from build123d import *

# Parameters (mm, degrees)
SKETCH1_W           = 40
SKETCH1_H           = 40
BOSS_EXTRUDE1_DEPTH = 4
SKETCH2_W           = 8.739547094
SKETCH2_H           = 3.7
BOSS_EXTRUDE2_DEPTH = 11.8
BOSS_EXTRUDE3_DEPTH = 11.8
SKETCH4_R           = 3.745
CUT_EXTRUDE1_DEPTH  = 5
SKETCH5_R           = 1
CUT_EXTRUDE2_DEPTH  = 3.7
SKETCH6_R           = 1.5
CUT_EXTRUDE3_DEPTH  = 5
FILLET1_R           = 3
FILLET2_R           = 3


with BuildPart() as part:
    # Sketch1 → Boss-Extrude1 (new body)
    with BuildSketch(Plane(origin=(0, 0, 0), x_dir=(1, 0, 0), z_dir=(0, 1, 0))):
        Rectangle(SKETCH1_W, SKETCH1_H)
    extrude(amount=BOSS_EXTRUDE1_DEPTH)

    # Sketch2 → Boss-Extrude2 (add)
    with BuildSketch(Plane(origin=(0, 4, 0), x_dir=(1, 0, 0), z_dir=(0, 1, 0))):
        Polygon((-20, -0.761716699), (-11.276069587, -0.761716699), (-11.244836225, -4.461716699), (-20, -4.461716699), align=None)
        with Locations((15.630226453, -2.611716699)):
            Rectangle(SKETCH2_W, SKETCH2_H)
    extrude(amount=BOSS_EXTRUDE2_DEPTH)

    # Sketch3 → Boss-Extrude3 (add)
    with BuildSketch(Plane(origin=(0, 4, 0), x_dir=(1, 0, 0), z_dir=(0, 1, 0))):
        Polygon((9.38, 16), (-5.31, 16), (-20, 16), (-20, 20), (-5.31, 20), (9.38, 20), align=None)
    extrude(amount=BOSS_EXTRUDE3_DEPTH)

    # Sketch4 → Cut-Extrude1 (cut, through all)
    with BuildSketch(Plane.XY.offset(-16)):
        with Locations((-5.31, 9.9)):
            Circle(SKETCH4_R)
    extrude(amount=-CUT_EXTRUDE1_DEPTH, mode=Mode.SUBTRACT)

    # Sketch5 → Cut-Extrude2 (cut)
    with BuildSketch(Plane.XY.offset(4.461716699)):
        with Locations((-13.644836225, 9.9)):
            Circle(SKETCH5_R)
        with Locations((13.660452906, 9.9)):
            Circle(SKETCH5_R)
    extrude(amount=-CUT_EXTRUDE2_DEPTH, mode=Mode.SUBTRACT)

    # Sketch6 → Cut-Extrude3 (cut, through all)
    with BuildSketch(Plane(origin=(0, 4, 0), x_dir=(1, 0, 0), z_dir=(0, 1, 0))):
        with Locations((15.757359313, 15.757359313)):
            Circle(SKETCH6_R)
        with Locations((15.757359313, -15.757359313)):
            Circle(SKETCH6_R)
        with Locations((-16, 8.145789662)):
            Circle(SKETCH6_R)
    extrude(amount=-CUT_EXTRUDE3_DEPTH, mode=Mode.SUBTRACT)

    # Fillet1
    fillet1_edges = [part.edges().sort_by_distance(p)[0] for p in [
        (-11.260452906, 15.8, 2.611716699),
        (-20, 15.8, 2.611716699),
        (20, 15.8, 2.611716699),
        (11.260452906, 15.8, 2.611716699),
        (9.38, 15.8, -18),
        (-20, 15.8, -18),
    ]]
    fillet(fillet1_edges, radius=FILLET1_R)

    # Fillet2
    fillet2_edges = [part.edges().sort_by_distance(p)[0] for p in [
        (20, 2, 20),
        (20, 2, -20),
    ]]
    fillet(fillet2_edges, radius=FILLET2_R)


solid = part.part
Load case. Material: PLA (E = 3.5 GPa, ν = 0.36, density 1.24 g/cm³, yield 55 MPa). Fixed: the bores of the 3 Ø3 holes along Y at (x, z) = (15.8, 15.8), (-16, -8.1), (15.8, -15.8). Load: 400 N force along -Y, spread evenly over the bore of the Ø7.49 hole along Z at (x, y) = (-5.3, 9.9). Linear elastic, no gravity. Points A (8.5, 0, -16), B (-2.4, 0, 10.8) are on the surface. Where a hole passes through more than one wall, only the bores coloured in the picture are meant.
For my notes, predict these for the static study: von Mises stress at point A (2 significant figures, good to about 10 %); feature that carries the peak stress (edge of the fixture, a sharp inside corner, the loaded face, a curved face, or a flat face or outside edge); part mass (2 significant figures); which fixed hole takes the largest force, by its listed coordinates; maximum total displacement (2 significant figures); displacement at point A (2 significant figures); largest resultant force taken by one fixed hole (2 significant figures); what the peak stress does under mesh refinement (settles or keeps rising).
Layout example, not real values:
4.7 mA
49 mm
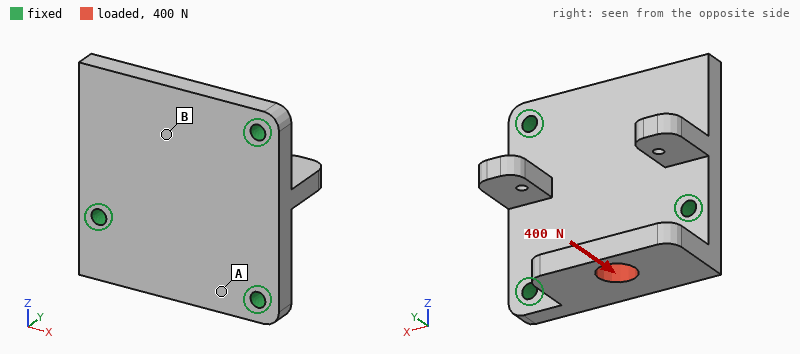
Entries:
14 MPa
edge of the fixture
10 g
(-16, -8.1)
0.57 mm
0.097 mm
260 N
keeps rising
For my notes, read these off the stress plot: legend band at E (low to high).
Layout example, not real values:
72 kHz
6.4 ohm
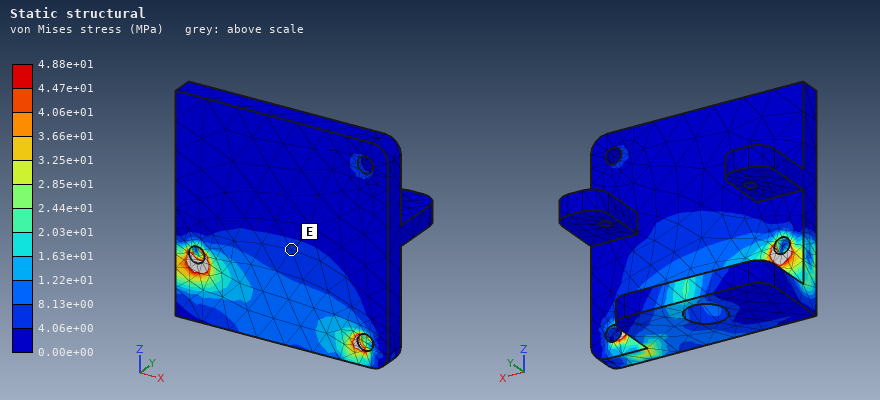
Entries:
4.06e+00 to 8.13e+00 MPa
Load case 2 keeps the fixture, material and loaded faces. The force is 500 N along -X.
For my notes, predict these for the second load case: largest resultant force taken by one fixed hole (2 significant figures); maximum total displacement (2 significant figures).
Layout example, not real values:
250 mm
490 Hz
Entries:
290 N
0.32 mm
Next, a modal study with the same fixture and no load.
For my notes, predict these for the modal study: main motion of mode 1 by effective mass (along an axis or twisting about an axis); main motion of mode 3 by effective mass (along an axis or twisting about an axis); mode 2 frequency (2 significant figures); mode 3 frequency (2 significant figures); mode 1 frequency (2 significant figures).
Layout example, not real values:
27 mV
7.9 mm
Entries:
along Y
along Y
3000 Hz
4300 Hz
2000 Hz
